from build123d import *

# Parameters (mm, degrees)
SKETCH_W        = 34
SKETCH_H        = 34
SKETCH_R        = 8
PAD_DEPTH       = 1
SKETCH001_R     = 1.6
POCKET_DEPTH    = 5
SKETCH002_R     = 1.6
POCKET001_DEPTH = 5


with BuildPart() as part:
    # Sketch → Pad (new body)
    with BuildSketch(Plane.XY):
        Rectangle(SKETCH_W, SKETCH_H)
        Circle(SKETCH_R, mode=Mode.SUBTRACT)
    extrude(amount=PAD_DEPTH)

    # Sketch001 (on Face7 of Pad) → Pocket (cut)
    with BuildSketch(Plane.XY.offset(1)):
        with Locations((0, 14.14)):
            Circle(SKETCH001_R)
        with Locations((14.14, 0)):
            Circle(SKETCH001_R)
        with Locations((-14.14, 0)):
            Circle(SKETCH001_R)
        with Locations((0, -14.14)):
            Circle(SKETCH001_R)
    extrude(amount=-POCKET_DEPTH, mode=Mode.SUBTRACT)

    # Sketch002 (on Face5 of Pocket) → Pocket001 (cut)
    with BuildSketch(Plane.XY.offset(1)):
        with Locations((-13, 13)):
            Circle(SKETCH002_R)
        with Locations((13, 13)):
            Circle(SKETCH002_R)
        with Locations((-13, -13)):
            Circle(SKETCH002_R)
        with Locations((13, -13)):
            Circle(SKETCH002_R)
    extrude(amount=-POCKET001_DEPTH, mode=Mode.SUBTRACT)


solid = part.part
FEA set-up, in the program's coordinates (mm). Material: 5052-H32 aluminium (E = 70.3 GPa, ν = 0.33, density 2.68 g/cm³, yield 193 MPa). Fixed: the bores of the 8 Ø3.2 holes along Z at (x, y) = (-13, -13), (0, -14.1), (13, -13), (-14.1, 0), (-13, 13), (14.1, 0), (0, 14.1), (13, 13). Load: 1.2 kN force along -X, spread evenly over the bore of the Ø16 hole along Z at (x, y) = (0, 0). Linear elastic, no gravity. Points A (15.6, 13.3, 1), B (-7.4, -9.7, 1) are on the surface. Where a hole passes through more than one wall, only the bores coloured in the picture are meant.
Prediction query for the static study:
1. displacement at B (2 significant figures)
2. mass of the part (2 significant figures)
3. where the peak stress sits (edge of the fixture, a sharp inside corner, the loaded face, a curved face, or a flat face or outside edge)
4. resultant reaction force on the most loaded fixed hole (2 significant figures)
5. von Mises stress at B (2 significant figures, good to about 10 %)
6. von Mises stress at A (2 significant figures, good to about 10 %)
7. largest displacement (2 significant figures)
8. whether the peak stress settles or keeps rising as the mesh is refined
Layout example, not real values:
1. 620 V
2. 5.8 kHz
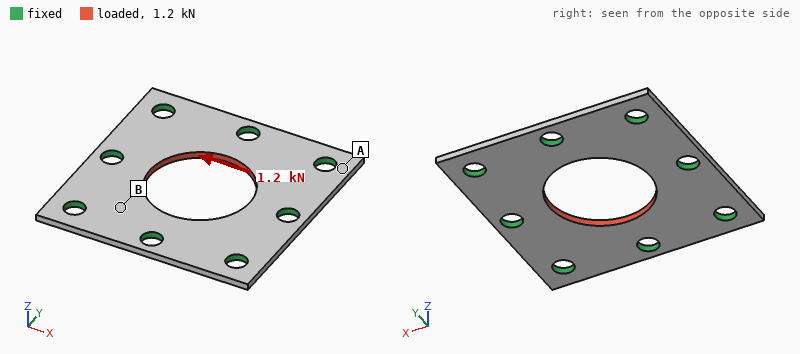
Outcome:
1. 1.5 µm
2. 2.4 g
3. edge of the fixture
4. 260 N
5. 20 MPa
6. 5.1 MPa
7. 3.5 µm
8. keeps rising
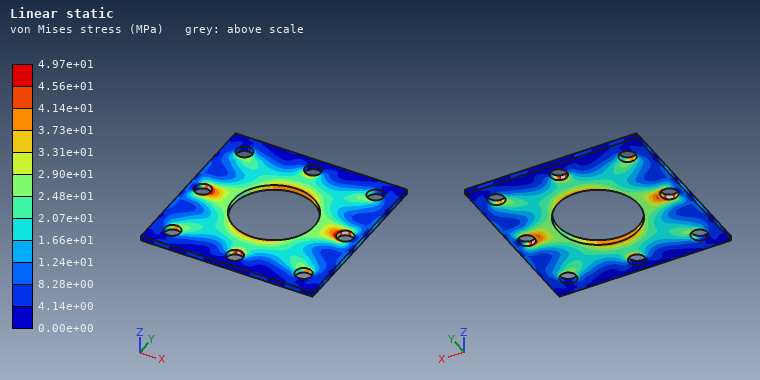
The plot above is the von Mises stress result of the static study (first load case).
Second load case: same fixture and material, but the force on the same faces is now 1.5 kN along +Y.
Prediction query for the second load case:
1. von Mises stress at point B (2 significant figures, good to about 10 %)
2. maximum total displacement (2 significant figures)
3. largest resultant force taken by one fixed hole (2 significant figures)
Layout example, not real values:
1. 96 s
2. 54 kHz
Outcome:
1. 21 MPa
2. 4.4 µm
3. 320 N
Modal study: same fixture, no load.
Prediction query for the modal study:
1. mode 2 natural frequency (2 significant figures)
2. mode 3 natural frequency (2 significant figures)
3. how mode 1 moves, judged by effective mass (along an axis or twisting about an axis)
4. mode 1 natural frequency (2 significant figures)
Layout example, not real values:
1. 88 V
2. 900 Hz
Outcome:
1. 24 kHz
2. 24 kHz
3. along Z
4. 22 kHz
